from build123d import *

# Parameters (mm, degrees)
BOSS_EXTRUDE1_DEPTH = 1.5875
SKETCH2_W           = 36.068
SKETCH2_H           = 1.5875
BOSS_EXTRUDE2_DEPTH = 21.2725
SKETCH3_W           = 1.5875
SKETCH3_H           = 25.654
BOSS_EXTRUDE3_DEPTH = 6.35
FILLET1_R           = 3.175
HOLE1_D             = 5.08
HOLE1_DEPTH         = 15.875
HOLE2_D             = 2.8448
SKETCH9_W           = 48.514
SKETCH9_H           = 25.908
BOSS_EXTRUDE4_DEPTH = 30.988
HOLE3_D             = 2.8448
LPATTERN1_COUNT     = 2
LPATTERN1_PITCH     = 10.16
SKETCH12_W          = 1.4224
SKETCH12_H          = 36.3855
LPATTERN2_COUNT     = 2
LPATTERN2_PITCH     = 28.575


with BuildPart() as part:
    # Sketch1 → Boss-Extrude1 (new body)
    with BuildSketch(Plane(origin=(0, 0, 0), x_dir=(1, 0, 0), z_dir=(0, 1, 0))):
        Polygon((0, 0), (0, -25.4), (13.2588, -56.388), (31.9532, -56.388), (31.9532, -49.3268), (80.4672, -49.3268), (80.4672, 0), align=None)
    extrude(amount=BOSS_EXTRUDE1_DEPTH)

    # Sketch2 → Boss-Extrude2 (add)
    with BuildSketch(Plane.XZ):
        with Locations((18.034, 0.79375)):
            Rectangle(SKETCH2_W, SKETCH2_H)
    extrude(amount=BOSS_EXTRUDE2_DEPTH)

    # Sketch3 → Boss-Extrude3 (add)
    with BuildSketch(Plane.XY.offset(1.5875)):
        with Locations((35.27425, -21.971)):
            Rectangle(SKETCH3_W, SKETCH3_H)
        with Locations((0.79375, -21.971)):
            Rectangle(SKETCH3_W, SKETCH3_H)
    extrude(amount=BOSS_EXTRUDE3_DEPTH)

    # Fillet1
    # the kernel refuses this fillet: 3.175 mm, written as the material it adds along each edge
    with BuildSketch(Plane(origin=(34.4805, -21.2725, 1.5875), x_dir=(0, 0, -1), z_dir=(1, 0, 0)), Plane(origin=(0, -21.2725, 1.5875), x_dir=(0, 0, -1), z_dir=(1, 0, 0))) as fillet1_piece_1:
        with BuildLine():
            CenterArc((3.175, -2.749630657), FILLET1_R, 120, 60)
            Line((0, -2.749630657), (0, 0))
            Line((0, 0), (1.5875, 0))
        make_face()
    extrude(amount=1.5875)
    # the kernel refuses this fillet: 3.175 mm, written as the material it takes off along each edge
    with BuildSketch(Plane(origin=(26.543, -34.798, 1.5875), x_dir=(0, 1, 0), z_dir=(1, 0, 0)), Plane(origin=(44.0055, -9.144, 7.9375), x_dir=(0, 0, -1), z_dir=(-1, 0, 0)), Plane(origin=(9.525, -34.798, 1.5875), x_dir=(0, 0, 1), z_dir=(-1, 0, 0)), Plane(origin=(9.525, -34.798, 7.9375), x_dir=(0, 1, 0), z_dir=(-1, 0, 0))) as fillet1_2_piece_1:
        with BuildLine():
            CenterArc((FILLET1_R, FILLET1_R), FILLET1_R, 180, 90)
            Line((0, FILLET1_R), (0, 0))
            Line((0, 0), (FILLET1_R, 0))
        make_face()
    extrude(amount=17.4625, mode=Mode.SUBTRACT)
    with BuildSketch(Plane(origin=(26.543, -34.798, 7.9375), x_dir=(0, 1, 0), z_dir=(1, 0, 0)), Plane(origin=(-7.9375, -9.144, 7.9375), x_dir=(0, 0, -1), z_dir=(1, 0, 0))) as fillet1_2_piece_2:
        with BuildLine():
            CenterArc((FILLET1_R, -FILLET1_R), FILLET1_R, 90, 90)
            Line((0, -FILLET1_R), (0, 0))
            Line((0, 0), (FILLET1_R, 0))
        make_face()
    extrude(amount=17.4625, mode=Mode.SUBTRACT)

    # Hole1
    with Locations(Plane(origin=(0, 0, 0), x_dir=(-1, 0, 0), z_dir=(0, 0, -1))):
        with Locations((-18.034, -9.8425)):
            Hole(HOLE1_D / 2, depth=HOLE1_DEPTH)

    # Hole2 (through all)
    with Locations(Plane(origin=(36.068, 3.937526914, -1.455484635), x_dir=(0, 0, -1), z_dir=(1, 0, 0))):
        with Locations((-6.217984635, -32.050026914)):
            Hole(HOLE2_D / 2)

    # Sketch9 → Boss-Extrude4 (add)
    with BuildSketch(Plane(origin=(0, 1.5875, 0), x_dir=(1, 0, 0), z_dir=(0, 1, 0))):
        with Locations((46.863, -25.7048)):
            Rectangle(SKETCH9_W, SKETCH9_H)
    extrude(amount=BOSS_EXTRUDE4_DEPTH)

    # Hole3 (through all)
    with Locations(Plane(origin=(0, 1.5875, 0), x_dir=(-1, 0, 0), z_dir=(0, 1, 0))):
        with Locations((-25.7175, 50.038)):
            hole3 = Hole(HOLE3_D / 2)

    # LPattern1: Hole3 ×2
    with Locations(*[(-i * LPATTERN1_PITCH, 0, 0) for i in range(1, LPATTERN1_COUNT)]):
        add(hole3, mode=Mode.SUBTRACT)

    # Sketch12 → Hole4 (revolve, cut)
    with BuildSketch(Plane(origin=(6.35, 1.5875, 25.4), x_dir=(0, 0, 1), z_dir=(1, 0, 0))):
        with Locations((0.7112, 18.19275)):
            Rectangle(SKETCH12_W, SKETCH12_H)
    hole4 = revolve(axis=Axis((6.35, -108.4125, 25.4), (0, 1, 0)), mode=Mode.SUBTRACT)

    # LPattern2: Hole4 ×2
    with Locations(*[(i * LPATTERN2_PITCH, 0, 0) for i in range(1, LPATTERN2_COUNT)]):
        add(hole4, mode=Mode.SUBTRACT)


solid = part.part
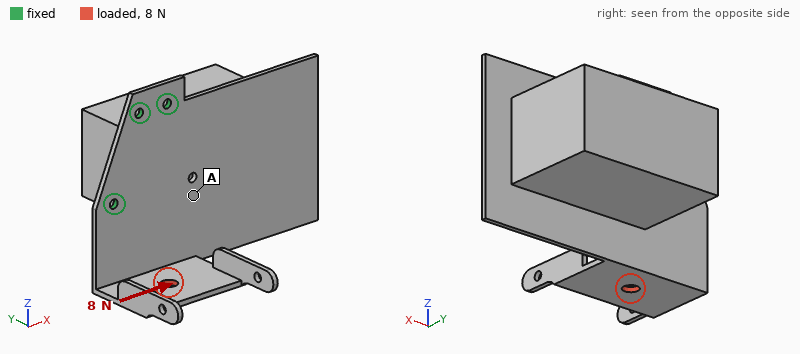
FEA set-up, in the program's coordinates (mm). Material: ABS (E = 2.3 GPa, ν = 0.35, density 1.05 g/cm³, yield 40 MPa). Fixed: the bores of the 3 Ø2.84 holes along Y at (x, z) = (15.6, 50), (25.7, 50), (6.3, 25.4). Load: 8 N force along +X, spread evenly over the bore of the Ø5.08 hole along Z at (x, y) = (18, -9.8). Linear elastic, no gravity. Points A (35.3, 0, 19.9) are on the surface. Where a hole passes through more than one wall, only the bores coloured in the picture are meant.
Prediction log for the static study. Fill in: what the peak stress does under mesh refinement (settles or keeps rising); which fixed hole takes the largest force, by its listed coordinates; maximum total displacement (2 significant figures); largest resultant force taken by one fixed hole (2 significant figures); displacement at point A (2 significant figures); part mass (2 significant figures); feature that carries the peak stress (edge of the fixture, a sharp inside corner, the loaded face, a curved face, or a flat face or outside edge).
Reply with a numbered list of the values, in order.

1. keeps rising
2. (6.3, 25.4)
3. 1.2 mm
4. 13 N
5. 0.36 mm
6. 49 g
7. edge of the fixture
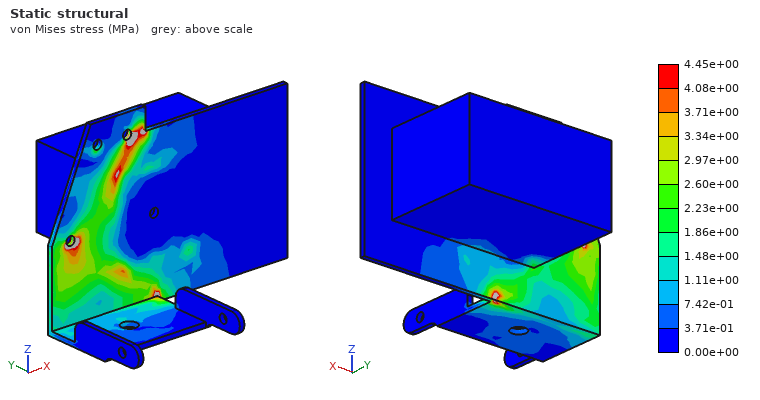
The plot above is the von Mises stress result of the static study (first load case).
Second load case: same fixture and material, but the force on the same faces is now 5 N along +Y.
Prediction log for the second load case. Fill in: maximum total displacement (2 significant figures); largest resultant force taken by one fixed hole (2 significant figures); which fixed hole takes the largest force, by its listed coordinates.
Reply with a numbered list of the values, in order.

1. 1.4 mm
2. 7.5 N
3. (6.3, 25.4)
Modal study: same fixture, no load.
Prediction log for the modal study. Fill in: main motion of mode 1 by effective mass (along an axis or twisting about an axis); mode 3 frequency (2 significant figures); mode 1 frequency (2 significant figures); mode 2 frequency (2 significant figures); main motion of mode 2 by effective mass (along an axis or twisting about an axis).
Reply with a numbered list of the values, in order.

1. along Y
2. 280 Hz
3. 43 Hz
4. 160 Hz
5. along Z
